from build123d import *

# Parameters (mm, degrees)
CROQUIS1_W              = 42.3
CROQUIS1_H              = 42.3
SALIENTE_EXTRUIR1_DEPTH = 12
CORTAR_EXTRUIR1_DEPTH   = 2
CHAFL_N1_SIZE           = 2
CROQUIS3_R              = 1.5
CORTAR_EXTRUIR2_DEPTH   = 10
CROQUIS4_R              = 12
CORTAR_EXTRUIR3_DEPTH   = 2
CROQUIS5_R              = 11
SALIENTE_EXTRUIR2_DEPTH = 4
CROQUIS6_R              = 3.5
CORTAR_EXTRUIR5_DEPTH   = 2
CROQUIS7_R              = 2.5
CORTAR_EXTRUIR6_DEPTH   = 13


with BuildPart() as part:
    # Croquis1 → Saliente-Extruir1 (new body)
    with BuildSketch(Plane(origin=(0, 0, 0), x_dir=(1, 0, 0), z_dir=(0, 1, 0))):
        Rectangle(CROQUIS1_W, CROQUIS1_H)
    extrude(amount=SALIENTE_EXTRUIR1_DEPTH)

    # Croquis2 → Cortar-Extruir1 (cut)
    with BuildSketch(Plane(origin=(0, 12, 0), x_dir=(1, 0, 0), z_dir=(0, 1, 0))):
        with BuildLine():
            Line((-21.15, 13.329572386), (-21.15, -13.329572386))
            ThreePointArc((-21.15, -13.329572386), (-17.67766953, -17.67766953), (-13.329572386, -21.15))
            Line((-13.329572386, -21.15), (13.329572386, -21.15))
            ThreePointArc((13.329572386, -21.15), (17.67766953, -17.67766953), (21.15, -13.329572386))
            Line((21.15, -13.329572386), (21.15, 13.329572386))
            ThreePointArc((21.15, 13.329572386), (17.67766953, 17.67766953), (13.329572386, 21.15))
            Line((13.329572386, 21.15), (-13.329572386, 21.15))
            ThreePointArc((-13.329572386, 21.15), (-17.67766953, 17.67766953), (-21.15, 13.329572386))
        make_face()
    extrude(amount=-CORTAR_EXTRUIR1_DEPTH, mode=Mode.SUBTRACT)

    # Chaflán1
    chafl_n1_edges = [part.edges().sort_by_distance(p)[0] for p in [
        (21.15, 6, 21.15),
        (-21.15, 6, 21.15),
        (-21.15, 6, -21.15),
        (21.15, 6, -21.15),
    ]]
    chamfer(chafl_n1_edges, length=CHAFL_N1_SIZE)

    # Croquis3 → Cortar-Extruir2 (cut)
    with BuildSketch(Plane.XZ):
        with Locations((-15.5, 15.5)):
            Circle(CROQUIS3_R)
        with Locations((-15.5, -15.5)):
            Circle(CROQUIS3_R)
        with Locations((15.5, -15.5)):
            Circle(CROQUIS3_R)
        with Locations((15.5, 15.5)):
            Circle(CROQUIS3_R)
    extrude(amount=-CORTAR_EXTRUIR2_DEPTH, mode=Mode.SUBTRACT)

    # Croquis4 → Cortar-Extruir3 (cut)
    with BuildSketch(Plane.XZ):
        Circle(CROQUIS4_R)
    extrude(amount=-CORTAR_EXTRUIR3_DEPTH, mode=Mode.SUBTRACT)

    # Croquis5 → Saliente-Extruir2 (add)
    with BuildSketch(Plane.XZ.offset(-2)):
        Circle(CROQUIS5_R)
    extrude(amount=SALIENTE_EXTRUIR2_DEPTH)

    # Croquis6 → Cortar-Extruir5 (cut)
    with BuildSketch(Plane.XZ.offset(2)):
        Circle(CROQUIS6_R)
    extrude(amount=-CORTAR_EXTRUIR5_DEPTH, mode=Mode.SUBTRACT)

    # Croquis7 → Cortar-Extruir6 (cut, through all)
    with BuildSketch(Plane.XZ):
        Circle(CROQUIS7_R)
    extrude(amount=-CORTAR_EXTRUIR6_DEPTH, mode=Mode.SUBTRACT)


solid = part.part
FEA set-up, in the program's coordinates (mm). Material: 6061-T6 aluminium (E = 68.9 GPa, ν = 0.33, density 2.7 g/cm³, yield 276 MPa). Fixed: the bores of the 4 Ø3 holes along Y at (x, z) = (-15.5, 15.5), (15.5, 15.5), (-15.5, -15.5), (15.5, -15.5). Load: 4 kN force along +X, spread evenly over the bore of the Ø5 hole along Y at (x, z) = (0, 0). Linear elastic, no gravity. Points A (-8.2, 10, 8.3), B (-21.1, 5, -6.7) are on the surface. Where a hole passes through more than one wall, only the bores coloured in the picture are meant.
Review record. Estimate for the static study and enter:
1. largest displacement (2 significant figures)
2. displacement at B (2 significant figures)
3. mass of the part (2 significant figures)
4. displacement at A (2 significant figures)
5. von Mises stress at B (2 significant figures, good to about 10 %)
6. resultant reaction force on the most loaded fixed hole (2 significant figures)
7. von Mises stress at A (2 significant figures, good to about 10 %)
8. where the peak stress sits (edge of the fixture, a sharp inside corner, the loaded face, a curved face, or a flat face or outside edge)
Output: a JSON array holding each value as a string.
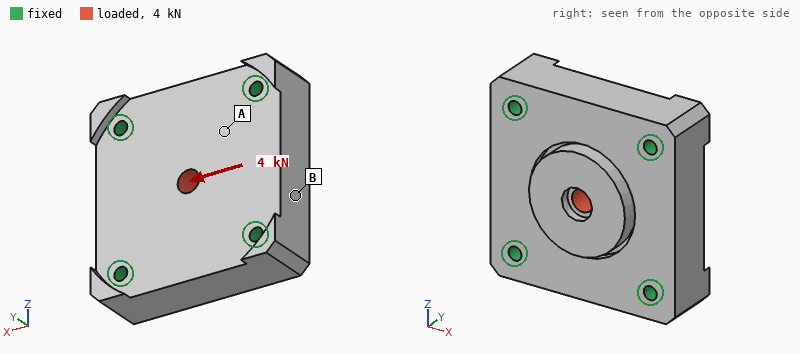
["4.9 µm", "2.1 µm", "49 g", "2.1 µm", "5.3 MPa", "1.1 kN", "11 MPa", "a sharp inside corner"]
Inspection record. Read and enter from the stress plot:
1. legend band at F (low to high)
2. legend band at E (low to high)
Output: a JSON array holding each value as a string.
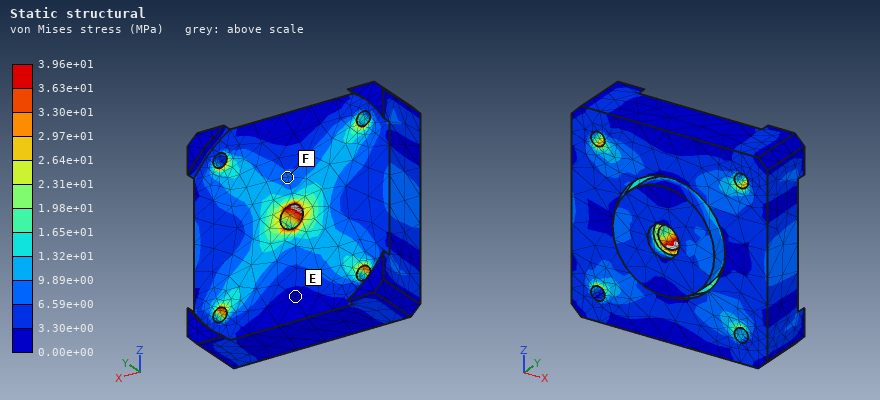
["6.59e+00 to 9.89e+00 MPa", "0.00e+00 to 3.30e+00 MPa"]
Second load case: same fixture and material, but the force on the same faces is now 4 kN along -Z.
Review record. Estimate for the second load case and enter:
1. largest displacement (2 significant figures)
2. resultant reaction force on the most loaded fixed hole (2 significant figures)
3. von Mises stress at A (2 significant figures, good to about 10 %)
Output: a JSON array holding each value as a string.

["4.9 µm", "1.1 kN", "11 MPa"]
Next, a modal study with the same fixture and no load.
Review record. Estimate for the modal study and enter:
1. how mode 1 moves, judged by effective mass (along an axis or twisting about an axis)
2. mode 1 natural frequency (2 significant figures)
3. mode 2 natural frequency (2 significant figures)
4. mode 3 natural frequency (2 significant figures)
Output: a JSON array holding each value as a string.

["along Y", "24 kHz", "34 kHz", "34 kHz"]
